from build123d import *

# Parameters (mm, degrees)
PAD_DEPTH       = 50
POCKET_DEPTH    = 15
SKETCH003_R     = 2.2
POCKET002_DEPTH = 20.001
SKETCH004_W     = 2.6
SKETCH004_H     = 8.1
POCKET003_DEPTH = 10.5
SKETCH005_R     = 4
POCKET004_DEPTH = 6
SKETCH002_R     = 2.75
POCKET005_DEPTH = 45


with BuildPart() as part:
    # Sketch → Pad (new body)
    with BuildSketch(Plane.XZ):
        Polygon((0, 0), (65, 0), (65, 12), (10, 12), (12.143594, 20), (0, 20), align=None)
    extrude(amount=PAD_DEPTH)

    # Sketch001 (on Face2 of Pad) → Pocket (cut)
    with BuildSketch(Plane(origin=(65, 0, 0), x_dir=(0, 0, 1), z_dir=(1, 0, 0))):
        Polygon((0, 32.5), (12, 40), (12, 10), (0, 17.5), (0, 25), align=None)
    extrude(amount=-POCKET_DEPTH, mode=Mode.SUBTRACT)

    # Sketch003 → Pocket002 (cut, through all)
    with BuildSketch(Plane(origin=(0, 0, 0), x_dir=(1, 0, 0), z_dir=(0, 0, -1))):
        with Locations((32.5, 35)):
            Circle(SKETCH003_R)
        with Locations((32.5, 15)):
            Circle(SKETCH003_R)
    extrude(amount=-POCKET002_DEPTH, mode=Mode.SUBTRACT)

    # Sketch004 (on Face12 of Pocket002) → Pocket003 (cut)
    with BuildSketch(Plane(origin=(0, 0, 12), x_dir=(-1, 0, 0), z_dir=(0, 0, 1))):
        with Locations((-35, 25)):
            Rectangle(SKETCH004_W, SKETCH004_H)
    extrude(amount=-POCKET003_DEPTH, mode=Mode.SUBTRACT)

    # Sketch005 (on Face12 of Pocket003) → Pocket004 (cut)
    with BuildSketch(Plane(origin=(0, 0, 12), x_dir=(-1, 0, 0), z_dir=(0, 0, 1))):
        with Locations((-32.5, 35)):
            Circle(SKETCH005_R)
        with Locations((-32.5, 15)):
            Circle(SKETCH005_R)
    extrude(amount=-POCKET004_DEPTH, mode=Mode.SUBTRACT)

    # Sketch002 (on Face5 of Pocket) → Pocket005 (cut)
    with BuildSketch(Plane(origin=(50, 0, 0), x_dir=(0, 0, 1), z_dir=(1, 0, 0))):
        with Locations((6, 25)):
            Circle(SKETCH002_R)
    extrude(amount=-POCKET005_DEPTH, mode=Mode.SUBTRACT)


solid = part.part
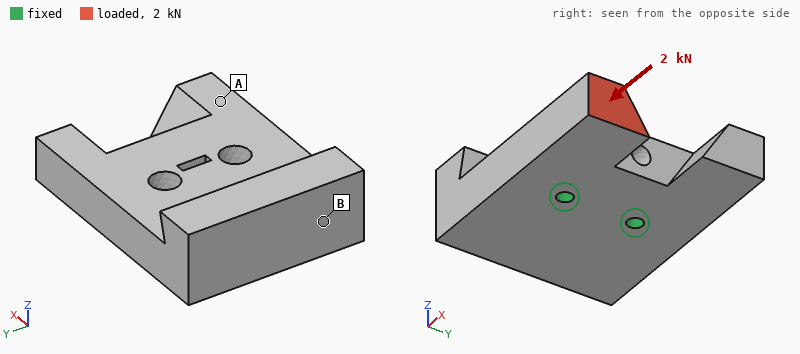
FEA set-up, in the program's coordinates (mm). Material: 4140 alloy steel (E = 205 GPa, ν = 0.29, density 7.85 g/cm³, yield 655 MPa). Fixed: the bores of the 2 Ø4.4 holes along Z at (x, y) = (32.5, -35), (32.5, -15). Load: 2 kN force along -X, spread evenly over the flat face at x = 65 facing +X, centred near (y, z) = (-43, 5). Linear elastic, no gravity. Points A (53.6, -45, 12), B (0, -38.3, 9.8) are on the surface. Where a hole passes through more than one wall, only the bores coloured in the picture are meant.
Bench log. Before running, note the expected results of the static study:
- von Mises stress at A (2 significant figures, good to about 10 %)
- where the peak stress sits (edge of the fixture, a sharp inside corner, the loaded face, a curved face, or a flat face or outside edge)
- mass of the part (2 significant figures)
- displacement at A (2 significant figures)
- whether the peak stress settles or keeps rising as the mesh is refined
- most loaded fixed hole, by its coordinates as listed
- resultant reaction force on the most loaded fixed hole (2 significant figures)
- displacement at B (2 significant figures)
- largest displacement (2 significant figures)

11 MPa
edge of the fixture
290 g
4.9 µm
keeps rising
(32.5, -35)
2.6 kN
4.1 µm
7.3 µm
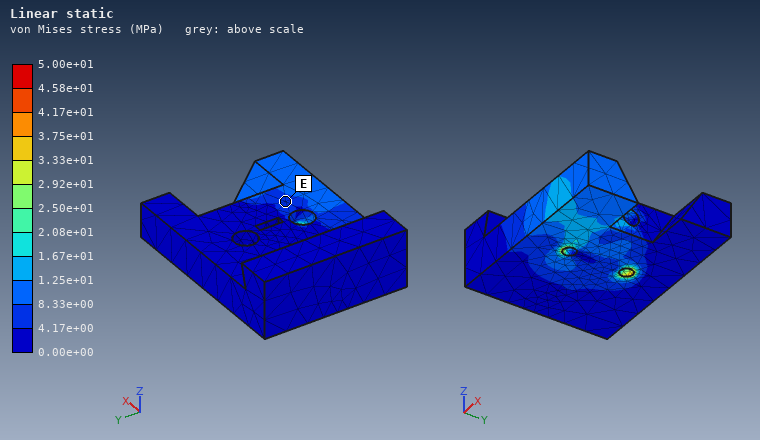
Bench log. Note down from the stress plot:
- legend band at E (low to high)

4.17e+00 to 8.33e+00 MPa
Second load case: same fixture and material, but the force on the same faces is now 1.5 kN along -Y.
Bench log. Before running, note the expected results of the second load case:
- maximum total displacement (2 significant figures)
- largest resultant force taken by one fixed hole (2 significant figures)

20 µm
2.2 kN
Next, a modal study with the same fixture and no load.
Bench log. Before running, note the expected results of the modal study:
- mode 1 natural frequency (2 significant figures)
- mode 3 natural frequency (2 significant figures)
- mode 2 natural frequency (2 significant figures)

3200 Hz
7900 Hz
7500 Hz
